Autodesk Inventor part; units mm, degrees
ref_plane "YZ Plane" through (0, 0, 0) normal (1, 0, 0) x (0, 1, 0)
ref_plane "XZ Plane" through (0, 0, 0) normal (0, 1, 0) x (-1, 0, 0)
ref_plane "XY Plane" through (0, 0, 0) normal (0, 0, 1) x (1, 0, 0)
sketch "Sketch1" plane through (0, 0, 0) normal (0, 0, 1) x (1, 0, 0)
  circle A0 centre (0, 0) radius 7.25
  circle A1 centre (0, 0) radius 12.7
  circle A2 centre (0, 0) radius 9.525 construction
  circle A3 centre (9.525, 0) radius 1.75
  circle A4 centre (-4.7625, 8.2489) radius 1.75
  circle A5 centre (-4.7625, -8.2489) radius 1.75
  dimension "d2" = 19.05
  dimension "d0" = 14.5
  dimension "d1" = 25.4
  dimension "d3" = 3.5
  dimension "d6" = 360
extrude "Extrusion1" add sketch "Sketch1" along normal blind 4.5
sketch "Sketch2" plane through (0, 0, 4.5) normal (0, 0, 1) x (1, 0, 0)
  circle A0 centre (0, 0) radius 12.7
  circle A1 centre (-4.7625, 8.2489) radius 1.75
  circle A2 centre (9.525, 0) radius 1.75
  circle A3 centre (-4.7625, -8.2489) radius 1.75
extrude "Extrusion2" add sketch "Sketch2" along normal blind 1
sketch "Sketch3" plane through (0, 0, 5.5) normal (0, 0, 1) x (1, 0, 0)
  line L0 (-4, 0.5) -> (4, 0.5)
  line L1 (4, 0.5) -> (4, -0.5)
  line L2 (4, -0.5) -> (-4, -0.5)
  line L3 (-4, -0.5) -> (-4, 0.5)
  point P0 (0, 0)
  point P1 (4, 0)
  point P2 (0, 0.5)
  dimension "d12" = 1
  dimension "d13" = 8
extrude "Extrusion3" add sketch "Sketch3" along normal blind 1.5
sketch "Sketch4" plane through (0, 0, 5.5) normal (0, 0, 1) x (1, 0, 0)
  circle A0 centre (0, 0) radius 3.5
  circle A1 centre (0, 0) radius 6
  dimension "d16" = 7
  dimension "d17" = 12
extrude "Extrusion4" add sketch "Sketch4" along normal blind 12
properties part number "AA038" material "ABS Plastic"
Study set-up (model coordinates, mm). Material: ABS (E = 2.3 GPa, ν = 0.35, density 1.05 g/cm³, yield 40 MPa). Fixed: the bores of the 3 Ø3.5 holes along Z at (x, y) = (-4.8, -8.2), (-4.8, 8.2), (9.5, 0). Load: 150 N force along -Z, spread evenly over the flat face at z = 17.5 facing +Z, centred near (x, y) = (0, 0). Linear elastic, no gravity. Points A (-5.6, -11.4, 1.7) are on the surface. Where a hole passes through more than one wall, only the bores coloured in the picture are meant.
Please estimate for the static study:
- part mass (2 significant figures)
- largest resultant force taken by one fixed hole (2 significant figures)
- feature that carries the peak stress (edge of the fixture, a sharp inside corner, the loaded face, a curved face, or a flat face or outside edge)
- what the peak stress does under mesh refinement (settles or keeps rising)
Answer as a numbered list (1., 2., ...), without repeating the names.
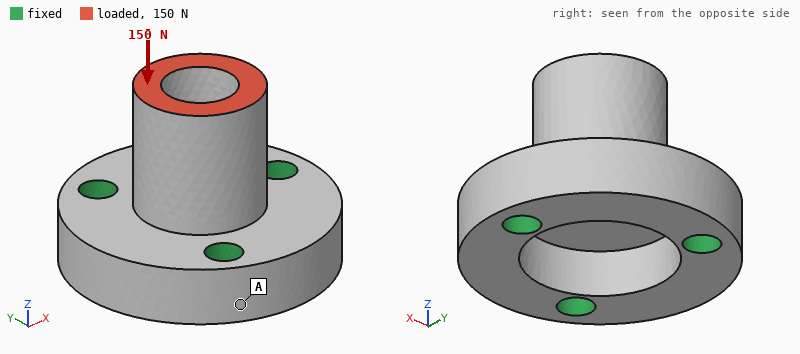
1. 2.9 g
2. 53 N
3. a sharp inside corner
4. keeps rising
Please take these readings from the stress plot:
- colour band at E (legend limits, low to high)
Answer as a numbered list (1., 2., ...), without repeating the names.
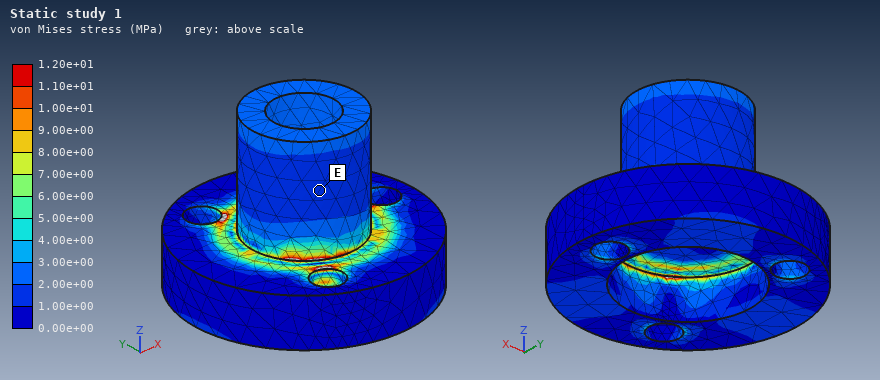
1. 1.00e+00 to 2.00e+00 MPa
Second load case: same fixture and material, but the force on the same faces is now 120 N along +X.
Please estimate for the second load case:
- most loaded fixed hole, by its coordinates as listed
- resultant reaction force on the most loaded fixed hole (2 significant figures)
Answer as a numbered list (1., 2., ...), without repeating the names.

1. (9.5, 0)
2. 120 N
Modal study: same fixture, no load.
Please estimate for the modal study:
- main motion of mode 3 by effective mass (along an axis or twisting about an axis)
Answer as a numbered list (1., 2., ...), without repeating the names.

1. along Z
